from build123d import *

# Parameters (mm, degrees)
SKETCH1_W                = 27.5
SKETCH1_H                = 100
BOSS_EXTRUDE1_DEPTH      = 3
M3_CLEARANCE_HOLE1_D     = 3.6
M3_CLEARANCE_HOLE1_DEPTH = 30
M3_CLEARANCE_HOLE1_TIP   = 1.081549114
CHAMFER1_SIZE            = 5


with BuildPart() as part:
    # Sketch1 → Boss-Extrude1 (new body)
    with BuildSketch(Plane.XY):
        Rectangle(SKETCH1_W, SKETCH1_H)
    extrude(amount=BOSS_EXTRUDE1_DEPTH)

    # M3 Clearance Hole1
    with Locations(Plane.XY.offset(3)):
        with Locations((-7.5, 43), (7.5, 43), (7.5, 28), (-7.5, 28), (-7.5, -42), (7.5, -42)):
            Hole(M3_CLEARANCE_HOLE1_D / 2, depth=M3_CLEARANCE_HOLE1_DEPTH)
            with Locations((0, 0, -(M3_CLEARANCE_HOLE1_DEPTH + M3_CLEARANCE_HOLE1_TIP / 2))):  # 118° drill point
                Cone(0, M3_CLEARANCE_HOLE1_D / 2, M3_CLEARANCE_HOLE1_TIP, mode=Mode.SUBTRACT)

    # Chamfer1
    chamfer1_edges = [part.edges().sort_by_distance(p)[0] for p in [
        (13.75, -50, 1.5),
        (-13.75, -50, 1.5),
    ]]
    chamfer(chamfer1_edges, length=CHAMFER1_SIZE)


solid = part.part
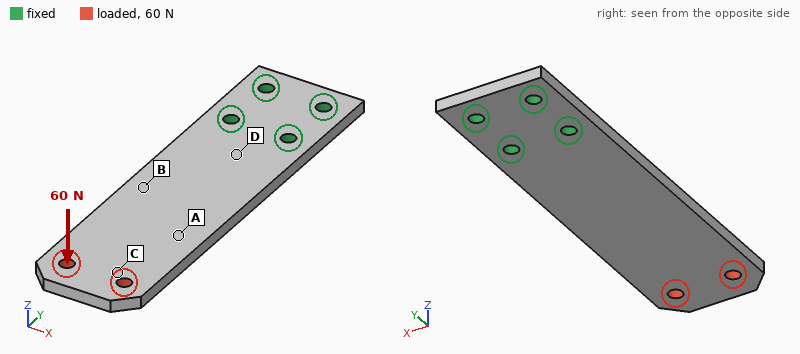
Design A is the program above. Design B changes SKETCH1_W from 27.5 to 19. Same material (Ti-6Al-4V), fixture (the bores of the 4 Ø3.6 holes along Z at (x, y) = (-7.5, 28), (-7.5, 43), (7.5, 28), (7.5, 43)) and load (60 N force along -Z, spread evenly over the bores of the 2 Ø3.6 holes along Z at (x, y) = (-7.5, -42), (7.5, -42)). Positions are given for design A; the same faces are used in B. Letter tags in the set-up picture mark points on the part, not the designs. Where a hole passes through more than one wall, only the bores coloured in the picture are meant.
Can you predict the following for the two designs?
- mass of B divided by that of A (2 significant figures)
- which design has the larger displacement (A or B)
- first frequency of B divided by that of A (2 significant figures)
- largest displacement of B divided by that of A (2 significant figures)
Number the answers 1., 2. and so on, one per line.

1. 0.68
2. B
3. 1.0
4. 1.5
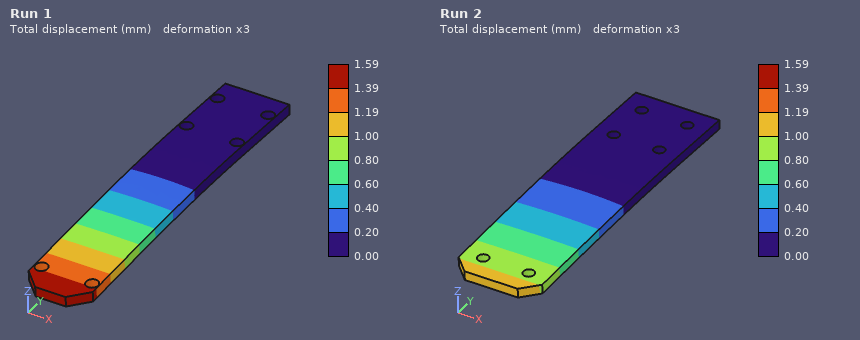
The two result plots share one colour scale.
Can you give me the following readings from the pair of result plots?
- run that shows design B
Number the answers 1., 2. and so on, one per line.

1. Run 1
